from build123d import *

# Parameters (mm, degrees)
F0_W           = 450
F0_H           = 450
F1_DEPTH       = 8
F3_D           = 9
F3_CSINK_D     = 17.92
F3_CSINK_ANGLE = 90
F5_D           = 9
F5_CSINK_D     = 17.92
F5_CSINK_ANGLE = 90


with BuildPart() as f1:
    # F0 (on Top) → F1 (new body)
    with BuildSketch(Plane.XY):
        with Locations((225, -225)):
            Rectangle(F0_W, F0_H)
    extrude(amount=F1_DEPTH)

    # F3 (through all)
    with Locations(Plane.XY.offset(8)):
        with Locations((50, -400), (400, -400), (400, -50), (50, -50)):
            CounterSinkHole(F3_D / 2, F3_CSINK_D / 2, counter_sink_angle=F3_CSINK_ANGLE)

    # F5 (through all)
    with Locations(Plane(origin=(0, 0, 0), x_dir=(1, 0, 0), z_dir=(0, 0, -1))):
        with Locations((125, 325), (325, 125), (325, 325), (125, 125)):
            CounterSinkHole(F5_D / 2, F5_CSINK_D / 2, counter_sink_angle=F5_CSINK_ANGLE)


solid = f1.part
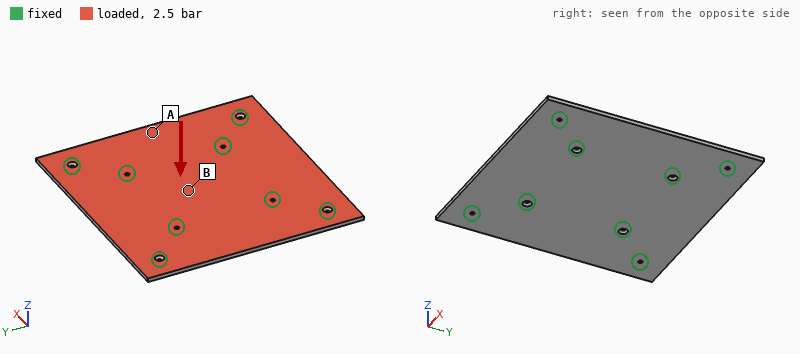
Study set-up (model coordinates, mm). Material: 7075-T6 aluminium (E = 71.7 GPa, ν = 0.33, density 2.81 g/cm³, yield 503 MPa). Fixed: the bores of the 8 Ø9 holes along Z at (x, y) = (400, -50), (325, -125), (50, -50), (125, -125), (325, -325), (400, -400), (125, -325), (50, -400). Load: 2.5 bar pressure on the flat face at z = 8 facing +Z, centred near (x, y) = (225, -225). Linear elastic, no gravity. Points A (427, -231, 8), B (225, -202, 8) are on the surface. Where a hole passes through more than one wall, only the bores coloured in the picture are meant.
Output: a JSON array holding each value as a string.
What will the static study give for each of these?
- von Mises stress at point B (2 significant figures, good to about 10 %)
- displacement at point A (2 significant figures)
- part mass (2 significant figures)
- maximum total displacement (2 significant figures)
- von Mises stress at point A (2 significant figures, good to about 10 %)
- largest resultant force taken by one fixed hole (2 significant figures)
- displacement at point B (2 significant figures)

["27 MPa", "1.5 mm", "4.5 kg", "1.8 mm", "55 MPa", "9.0 kN", "0.69 mm"]
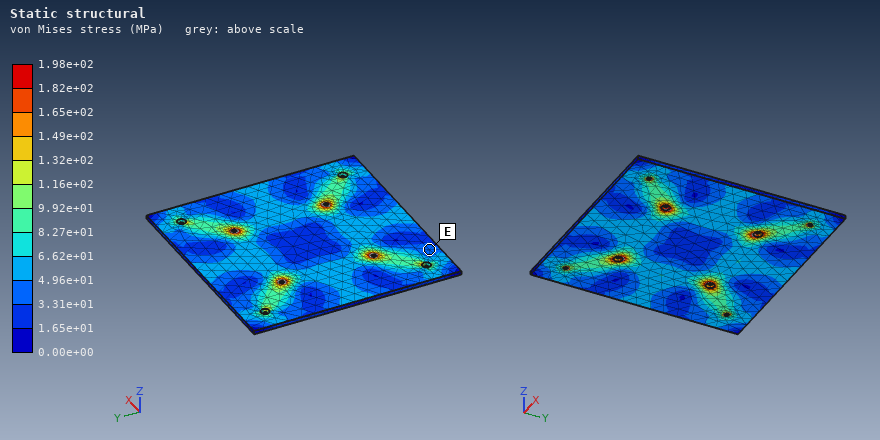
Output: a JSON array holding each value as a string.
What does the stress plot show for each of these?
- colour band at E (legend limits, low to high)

["3.31e+01 to 4.96e+01 MPa"]
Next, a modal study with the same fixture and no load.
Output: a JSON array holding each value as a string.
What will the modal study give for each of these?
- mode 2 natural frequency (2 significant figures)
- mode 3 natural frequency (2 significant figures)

["450 Hz", "450 Hz"]
